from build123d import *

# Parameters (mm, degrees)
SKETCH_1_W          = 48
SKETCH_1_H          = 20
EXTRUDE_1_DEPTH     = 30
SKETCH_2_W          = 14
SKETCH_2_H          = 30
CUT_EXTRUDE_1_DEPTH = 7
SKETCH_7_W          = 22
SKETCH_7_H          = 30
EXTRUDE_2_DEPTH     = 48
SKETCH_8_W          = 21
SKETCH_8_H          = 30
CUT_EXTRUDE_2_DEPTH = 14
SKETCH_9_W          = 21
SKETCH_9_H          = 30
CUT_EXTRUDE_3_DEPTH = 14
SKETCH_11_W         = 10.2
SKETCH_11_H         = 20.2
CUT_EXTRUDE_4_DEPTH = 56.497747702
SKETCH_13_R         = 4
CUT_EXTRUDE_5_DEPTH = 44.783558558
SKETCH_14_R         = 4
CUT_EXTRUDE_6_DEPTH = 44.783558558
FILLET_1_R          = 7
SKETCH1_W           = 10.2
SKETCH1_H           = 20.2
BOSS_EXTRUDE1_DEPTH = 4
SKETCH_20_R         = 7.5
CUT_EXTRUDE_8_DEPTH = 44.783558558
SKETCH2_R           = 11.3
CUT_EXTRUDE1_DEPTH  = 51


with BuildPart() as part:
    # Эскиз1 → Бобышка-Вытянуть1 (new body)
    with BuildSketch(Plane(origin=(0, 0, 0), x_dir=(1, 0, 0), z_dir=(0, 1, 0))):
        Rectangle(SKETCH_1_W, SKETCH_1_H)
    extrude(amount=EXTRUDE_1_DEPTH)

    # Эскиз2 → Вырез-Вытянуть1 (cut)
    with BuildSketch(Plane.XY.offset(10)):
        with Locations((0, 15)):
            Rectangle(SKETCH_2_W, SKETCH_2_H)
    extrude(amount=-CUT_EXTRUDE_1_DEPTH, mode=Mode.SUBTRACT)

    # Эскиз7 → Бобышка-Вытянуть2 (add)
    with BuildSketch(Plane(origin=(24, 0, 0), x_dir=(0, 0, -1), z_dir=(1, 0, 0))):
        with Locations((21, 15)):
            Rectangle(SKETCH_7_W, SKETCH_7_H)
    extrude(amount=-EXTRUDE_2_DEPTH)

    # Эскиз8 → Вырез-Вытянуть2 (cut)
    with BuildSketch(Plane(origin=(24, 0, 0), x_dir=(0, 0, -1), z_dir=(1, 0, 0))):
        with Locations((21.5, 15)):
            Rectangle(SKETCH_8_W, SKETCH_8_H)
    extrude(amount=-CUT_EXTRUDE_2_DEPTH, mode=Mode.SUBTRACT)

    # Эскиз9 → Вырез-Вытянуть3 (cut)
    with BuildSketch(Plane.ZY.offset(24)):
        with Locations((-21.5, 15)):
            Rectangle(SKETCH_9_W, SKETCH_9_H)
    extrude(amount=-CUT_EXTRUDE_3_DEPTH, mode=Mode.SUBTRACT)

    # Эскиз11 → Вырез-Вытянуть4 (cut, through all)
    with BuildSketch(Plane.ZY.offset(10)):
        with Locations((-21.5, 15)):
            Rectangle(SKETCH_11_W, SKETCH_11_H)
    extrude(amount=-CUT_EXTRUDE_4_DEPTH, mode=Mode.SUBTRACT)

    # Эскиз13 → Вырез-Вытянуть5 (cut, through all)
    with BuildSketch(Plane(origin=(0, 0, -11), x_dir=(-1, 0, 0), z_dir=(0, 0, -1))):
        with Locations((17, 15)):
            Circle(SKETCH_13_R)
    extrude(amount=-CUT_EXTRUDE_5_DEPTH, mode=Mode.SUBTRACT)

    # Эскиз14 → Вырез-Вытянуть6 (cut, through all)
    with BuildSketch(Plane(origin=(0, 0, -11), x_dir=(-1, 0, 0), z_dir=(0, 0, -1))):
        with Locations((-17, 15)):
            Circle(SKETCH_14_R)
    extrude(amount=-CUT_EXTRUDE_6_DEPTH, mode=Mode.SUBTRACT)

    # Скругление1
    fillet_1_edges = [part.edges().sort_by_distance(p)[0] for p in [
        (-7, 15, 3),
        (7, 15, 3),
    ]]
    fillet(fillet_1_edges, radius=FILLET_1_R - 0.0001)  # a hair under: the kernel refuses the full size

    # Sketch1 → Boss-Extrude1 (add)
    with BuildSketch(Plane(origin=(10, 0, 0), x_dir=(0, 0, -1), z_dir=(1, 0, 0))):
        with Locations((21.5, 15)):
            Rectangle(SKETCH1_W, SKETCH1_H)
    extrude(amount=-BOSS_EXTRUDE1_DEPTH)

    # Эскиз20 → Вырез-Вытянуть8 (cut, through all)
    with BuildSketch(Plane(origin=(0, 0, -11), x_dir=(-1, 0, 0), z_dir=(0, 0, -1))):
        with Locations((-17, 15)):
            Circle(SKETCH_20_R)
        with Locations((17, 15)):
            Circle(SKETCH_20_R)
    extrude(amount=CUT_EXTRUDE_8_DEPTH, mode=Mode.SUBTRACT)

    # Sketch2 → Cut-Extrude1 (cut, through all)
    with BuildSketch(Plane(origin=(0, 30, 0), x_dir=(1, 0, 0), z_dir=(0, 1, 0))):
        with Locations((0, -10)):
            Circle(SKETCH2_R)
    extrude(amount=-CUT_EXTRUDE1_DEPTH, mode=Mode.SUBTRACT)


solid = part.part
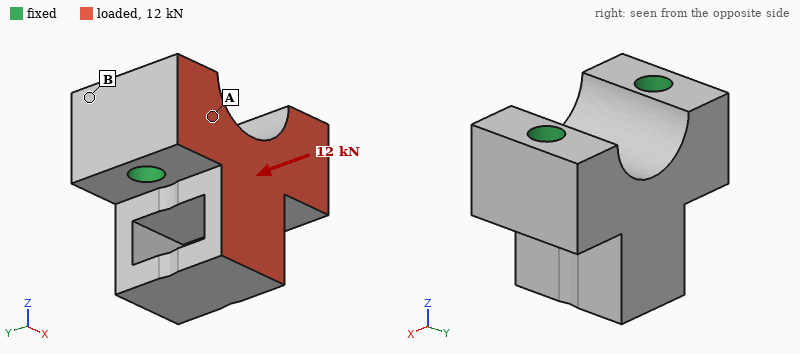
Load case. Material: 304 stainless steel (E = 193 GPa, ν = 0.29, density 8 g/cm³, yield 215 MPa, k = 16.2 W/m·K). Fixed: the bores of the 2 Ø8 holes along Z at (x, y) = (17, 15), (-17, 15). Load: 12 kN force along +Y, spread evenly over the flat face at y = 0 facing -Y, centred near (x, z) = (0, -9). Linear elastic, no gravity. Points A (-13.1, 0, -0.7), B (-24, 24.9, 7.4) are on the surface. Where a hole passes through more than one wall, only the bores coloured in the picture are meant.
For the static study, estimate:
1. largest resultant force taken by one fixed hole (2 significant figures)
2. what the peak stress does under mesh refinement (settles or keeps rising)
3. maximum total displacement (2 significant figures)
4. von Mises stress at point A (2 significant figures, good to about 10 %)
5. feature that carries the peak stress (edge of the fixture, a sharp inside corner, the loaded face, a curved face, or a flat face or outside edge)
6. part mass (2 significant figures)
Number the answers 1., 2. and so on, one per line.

1. 6.0 kN
2. keeps rising
3. 17 µm
4. 20 MPa
5. edge of the fixture
6. 250 g
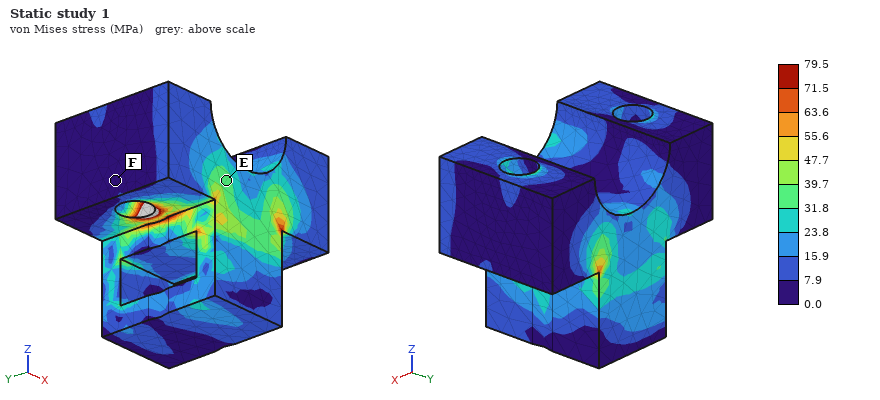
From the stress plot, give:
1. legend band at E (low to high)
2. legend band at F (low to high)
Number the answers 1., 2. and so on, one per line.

1. 31.8 to 39.7 MPa
2. 0.0 to 7.9 MPa
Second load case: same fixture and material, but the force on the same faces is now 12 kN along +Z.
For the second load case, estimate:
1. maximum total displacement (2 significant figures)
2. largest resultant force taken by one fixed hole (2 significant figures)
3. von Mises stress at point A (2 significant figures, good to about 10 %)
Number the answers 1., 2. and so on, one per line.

1. 16 µm
2. 6.2 kN
3. 30 MPa
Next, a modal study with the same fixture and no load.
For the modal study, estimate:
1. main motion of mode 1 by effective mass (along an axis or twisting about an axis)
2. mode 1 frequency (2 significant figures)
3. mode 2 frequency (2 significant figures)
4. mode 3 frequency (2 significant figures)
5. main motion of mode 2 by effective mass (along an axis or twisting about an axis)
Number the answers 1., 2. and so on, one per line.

1. along Y
2. 11 kHz
3. 14 kHz
4. 21 kHz
5. along X
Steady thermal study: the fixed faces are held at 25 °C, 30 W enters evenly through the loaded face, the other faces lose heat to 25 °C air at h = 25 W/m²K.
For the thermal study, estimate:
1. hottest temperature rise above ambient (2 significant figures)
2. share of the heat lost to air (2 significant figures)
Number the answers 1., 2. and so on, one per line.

1. 52 K
2. 9.4 %
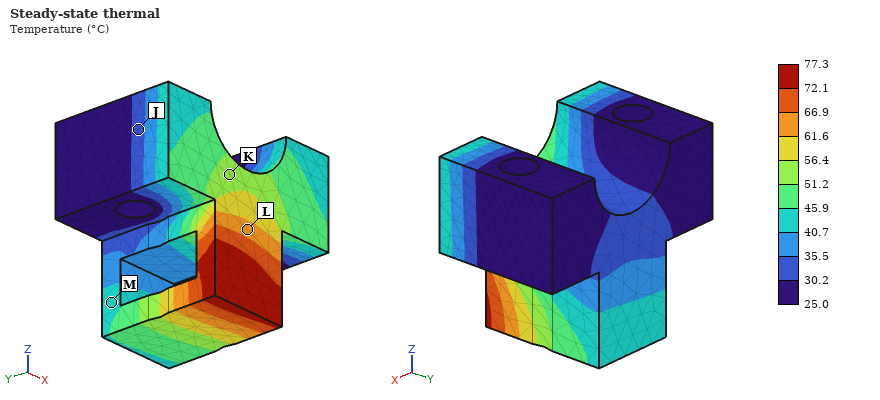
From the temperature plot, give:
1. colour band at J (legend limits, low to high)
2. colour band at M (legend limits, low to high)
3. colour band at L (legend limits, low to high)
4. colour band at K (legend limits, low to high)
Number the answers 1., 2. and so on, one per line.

1. 30.2 to 35.5 °C
2. 40.7 to 45.9 °C
3. 61.6 to 66.9 °C
4. 51.2 to 56.4 °C
